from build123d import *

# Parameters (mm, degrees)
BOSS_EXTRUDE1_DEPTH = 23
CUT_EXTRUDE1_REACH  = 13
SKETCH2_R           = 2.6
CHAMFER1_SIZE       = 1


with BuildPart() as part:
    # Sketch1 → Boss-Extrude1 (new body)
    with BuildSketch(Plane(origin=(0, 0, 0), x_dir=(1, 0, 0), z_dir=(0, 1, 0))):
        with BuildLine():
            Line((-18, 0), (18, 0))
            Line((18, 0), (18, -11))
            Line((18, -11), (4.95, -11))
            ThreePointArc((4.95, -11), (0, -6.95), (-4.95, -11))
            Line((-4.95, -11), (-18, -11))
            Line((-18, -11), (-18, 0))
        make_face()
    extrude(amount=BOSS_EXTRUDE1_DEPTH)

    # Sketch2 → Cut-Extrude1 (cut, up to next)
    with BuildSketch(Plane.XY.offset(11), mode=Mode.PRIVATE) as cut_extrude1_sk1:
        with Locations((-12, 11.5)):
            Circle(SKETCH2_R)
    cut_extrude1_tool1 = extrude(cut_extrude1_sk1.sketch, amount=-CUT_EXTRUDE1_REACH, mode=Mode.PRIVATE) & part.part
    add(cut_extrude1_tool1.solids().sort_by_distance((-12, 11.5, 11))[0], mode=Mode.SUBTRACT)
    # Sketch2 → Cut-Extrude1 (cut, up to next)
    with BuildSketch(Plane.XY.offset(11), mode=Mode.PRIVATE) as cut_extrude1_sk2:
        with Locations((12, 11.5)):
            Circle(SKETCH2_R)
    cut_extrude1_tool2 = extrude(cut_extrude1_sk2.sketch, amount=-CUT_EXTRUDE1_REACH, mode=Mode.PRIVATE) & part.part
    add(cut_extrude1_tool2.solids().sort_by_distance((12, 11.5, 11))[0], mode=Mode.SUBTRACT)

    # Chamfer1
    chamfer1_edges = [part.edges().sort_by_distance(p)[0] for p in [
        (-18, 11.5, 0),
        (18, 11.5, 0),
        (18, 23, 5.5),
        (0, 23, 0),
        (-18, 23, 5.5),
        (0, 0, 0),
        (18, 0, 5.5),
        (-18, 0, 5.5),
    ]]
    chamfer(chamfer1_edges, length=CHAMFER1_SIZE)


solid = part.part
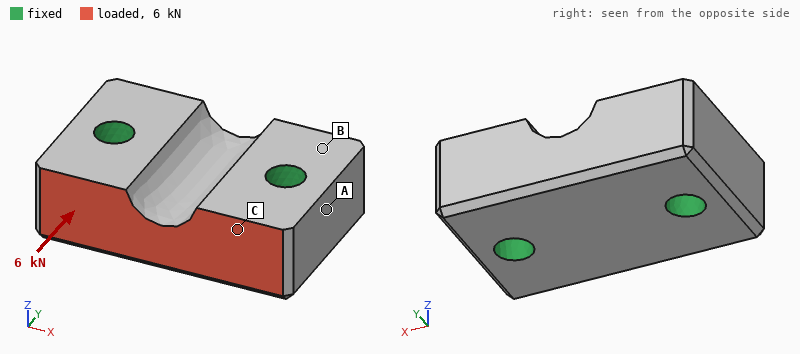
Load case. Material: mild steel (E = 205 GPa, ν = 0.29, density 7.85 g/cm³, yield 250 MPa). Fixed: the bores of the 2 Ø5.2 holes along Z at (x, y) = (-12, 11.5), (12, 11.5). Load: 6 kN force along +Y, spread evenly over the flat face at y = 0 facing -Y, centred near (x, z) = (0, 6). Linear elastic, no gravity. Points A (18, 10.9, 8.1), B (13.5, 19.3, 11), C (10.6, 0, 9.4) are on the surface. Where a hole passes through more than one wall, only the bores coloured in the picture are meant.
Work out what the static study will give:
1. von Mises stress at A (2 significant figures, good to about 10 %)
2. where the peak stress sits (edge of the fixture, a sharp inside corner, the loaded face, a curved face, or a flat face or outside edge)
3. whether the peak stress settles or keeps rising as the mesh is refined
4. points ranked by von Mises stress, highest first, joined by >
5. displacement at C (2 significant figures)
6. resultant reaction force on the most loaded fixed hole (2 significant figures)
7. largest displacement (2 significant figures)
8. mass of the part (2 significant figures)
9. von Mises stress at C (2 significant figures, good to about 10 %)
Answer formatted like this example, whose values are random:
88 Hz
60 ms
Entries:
8.9 MPa
edge of the fixture
keeps rising
C > A > B
1.2 µm
3.0 kN
1.5 µm
62 g
20 MPa
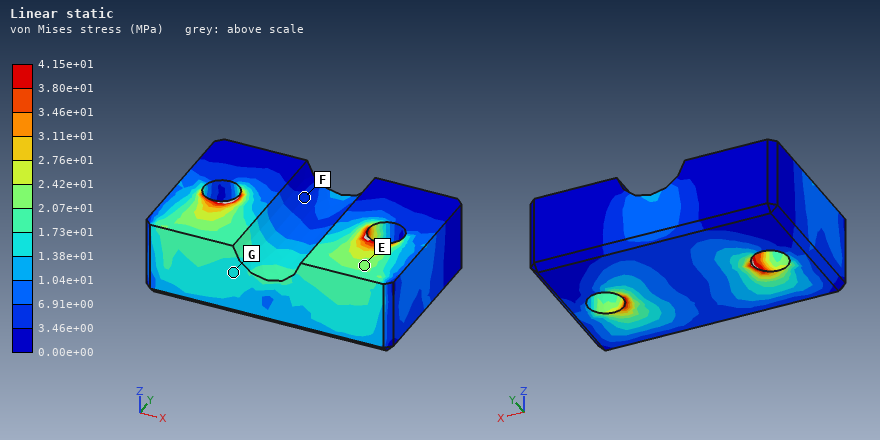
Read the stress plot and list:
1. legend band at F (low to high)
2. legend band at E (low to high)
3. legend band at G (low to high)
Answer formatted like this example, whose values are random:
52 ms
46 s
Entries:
3.46e+00 to 6.91e+00 MPa
2.07e+01 to 2.42e+01 MPa
1.38e+01 to 1.73e+01 MPa
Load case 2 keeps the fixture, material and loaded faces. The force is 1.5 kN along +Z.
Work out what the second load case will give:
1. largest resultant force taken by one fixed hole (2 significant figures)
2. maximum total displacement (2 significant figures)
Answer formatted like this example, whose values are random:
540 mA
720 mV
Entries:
750 N
2.2 µm
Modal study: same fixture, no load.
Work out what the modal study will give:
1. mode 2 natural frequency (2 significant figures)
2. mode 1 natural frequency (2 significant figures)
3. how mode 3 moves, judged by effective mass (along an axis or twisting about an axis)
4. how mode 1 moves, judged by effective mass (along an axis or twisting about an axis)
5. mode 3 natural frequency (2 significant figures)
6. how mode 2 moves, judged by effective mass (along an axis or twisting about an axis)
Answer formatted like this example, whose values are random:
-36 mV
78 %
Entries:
45 kHz
42 kHz
along Y
twisting about X
54 kHz
along Z
